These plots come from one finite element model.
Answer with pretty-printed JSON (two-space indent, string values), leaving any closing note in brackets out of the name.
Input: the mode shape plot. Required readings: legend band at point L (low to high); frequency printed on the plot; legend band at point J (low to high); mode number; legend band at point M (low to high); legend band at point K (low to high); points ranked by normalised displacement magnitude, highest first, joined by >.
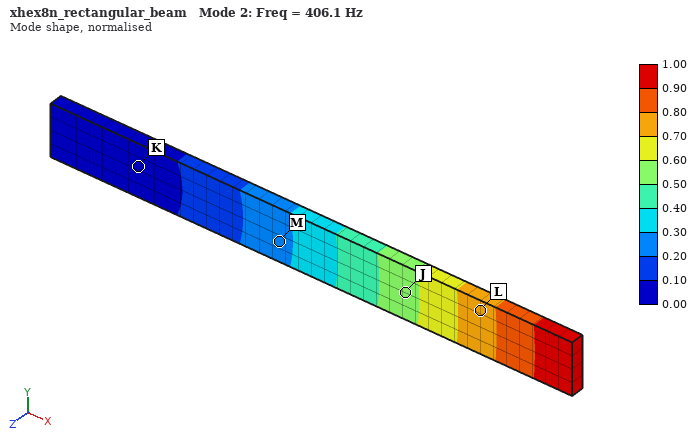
{
  "legend band at point L": "0.70 to 0.80",
  "frequency printed on the plot": "406.1 Hz",
  "legend band at point J": "0.50 to 0.60",
  "mode number": "2",
  "legend band at point M": "0.20 to 0.30",
  "legend band at point K": "0.00 to 0.10",
  "points ranked by normalised displacement magnitude, highest first, joined by >": "L > J > M > K"
}
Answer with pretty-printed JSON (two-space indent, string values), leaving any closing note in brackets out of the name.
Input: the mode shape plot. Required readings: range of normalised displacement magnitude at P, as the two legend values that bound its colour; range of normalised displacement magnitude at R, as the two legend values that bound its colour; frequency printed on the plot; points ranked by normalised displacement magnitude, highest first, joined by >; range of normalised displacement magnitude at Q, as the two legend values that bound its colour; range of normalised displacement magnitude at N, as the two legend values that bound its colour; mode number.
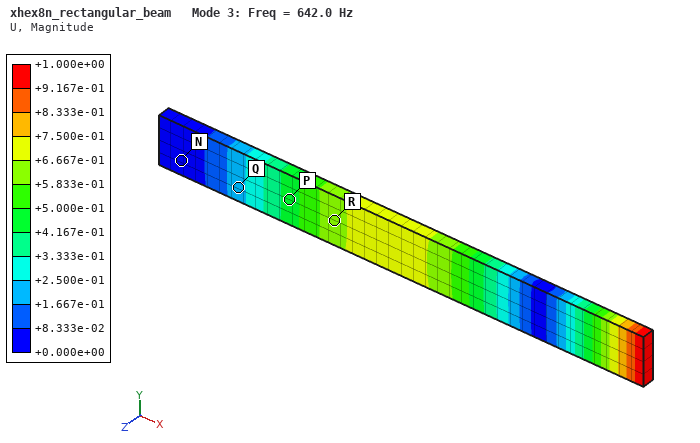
{
  "range of normalised displacement magnitude at P, as the two legend values that bound its colour": "+4.167e-01 to +5.000e-01",
  "range of normalised displacement magnitude at R, as the two legend values that bound its colour": "+5.833e-01 to +6.667e-01",
  "frequency printed on the plot": "642.0 Hz",
  "points ranked by normalised displacement magnitude, highest first, joined by >": "R > P > Q > N",
  "range of normalised displacement magnitude at Q, as the two legend values that bound its colour": "+1.667e-01 to +2.500e-01",
  "range of normalised displacement magnitude at N, as the two legend values that bound its colour": "+0.000e+00 to +8.333e-02",
  "mode number": "3"
}
